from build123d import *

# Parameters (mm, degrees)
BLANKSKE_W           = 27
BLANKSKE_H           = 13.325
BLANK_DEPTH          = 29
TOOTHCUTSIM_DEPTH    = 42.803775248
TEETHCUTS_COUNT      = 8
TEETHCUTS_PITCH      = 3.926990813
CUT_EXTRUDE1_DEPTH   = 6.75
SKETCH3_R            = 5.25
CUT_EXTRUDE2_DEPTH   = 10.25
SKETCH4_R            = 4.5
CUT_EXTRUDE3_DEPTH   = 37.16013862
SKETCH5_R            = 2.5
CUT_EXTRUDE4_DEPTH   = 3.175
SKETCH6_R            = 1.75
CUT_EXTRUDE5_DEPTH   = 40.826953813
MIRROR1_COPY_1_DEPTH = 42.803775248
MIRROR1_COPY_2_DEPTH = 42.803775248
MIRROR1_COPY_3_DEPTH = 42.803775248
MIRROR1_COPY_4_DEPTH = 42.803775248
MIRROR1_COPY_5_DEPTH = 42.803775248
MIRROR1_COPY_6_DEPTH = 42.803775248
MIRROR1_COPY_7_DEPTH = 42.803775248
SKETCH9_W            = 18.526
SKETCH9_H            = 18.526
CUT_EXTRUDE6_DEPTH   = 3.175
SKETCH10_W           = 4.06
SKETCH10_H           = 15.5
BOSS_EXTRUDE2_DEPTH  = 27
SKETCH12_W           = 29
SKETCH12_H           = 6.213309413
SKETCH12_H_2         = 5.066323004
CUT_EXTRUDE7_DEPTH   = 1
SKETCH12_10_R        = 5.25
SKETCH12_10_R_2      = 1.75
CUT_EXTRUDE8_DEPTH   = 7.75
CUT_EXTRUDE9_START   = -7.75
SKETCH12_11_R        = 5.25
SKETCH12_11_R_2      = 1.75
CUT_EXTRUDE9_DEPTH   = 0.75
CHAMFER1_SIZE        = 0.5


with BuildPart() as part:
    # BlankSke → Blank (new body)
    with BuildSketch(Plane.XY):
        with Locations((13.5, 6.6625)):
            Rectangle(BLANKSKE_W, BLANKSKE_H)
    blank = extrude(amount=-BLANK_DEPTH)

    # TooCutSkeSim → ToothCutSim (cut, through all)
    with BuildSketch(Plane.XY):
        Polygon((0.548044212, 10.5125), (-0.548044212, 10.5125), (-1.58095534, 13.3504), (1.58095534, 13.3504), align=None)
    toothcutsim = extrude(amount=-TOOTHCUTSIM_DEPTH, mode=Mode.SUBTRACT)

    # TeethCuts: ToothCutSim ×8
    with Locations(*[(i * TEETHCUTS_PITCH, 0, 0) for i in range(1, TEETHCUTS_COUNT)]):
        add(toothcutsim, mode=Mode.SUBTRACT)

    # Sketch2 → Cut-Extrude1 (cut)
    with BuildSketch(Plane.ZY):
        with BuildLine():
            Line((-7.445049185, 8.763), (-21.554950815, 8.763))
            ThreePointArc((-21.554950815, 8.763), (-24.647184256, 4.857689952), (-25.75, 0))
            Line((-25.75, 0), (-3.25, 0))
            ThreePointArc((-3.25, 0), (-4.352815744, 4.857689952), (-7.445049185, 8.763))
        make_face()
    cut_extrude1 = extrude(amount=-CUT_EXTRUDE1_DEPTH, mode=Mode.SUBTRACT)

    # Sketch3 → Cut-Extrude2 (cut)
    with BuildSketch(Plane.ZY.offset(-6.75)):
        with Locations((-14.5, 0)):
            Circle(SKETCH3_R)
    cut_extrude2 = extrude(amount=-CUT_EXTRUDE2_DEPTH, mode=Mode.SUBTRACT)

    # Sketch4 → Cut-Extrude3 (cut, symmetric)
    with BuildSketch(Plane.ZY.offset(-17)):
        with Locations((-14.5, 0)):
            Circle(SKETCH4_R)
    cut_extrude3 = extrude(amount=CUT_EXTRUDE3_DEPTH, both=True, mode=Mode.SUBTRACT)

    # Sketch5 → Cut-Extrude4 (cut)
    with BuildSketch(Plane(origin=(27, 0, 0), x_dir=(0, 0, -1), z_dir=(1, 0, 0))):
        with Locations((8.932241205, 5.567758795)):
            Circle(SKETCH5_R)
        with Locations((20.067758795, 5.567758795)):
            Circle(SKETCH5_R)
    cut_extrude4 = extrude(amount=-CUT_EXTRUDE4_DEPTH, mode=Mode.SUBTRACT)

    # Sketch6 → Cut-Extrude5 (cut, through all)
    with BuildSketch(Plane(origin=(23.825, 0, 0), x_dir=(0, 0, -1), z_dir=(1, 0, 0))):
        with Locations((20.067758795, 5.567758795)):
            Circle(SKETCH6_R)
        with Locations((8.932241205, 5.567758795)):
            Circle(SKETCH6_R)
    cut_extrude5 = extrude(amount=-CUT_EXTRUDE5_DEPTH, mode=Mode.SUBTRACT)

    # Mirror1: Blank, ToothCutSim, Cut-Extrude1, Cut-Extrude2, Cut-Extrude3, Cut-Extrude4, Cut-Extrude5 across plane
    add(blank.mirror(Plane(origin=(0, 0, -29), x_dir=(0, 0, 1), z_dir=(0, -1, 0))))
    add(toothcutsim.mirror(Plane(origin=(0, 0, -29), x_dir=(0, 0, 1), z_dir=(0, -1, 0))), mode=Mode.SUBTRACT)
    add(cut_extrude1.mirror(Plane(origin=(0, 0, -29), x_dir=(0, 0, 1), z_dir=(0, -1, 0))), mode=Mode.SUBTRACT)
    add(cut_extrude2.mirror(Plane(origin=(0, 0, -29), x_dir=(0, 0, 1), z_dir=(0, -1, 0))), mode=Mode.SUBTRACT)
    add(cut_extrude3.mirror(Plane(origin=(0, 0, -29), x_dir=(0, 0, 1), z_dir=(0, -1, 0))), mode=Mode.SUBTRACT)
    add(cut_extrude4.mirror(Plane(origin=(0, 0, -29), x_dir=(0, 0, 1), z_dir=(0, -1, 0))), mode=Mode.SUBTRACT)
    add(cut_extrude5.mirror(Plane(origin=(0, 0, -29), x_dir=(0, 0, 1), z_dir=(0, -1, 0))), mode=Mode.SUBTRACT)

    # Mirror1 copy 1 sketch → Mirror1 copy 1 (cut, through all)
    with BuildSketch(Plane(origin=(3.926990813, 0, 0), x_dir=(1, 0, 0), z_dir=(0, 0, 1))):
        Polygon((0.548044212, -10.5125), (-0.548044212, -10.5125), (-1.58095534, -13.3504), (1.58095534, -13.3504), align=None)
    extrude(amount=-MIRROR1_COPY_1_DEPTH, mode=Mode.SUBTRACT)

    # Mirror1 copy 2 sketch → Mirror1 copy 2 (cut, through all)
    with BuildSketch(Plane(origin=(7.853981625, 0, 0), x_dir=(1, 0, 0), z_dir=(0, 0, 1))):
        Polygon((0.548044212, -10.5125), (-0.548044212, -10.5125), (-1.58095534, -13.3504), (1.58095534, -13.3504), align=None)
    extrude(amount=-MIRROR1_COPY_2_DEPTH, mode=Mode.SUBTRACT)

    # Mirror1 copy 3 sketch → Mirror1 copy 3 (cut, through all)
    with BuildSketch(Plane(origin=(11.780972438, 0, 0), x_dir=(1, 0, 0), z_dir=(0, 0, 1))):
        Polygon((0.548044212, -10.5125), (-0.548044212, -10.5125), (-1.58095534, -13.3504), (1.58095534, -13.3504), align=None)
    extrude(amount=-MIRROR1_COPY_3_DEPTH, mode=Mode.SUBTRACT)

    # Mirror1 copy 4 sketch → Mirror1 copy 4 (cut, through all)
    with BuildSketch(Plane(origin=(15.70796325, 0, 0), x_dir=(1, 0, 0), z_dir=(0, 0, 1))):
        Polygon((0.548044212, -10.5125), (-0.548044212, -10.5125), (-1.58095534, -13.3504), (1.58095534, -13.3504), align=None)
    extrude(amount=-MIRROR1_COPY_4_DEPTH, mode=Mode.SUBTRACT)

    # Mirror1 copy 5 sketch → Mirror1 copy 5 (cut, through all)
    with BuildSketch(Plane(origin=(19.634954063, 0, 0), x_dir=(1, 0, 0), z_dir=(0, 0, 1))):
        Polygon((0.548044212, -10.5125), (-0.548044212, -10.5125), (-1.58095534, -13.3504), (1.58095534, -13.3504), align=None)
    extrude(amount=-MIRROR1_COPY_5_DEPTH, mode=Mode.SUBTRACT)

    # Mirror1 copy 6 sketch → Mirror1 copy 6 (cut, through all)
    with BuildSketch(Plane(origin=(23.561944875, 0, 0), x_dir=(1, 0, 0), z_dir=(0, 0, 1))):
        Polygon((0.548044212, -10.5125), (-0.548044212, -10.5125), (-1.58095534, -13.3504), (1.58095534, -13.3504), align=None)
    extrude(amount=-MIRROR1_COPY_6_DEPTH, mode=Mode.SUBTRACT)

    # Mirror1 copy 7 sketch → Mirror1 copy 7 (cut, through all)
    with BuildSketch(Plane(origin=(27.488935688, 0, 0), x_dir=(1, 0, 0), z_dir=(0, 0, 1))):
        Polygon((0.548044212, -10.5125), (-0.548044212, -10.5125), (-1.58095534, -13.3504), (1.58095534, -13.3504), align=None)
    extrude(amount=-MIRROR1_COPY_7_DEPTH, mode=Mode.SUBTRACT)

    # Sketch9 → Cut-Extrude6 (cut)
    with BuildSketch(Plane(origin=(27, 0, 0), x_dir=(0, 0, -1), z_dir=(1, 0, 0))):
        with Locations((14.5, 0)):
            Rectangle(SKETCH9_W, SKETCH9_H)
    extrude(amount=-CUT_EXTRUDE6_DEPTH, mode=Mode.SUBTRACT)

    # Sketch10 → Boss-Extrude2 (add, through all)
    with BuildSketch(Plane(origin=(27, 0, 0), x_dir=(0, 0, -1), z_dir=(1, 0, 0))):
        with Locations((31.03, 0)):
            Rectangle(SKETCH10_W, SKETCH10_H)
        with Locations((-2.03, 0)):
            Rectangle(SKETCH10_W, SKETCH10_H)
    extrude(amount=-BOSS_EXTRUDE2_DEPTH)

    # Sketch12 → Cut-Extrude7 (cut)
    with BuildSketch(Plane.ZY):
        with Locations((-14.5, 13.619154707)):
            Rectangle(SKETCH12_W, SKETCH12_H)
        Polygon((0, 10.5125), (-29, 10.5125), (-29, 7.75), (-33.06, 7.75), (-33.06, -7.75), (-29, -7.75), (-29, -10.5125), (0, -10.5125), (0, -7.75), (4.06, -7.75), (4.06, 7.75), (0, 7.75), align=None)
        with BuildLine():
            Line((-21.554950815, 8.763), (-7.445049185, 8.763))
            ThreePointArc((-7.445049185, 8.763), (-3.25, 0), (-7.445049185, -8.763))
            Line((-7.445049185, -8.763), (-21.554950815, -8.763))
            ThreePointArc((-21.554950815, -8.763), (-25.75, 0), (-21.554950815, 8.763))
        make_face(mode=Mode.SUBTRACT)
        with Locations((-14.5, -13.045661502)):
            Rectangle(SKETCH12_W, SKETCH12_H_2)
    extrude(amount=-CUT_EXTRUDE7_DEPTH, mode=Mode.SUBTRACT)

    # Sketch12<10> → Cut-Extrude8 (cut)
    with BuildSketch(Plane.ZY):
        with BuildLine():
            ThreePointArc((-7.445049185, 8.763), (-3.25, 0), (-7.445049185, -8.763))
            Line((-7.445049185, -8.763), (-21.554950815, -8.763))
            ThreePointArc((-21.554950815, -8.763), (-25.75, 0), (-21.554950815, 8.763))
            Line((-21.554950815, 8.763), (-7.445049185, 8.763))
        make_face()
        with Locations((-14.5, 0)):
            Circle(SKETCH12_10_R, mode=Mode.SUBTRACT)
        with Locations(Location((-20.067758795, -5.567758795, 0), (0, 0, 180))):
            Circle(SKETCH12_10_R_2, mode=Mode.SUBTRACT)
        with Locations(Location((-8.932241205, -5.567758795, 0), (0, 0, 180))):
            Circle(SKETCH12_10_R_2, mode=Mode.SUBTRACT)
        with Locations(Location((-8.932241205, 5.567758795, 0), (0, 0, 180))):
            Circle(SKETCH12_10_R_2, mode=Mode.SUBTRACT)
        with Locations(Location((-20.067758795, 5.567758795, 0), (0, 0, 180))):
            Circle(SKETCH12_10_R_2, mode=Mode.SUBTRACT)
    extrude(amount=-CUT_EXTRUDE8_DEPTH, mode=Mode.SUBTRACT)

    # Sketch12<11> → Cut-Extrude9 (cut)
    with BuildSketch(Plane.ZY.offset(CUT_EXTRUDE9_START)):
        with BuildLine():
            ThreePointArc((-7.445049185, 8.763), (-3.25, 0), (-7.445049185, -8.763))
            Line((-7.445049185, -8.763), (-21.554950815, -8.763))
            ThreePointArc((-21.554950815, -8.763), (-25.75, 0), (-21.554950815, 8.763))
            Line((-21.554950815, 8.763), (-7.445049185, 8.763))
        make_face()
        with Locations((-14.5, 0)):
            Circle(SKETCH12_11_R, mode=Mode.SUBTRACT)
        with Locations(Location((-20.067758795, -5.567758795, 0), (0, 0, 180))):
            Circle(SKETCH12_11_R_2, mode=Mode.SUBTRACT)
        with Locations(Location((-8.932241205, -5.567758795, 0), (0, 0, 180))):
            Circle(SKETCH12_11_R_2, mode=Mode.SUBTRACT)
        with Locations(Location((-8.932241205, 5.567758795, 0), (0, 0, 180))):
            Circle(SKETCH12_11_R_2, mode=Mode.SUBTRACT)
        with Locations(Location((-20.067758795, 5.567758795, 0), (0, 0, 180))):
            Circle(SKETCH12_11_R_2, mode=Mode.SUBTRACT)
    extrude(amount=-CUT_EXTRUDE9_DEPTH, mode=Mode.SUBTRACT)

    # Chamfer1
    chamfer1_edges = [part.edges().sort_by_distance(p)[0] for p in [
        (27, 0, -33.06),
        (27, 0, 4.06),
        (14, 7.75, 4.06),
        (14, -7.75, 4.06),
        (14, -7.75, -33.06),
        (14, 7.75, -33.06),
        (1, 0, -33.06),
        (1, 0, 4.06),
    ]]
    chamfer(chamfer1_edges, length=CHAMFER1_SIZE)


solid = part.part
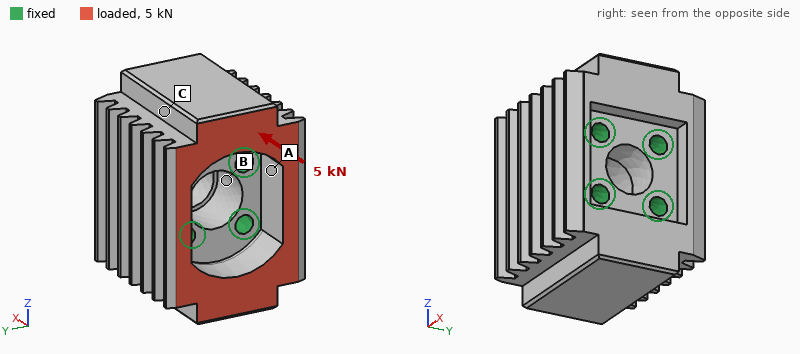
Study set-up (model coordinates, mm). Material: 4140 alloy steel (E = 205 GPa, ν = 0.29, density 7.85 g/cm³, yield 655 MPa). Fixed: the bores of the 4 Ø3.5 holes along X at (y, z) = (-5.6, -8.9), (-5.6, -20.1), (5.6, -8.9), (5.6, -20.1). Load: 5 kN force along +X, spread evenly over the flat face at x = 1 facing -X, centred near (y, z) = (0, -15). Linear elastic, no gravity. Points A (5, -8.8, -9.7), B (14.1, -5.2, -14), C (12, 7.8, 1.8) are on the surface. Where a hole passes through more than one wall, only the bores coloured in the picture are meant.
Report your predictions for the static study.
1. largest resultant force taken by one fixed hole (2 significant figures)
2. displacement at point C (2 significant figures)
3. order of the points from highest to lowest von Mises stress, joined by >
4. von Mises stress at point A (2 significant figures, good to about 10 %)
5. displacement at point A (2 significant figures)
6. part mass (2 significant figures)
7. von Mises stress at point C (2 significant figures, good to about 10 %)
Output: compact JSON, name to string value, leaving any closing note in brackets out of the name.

{"largest resultant force taken by one fixed hole": "1.3 kN", "displacement at point C": "0.99 µm", "order of the points from highest to lowest von Mises stress, joined by >": "A > C > B", "von Mises stress at point A": "15 MPa", "displacement at point A": "0.77 µm", "part mass": "120 g", "von Mises stress at point C": "8.6 MPa"}
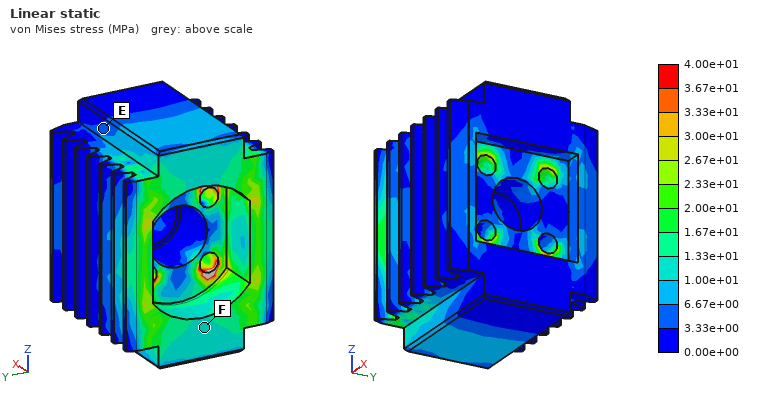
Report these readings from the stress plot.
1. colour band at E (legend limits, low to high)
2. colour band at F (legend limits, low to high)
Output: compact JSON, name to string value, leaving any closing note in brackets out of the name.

{"colour band at E": "3.33e+00 to 6.67e+00 MPa", "colour band at F": "1.00e+01 to 1.33e+01 MPa"}
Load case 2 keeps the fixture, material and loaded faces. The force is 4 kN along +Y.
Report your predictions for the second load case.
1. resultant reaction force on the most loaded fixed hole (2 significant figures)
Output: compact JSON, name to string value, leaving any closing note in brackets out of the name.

{"resultant reaction force on the most loaded fixed hole": "1.7 kN"}
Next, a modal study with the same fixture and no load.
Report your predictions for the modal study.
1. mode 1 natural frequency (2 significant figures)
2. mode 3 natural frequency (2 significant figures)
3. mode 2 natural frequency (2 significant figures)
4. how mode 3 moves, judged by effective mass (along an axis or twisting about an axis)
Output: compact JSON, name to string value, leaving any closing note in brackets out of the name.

{"mode 1 natural frequency": "32 kHz", "mode 3 natural frequency": "34 kHz", "mode 2 natural frequency": "32 kHz", "how mode 3 moves, judged by effective mass": "along X"}
